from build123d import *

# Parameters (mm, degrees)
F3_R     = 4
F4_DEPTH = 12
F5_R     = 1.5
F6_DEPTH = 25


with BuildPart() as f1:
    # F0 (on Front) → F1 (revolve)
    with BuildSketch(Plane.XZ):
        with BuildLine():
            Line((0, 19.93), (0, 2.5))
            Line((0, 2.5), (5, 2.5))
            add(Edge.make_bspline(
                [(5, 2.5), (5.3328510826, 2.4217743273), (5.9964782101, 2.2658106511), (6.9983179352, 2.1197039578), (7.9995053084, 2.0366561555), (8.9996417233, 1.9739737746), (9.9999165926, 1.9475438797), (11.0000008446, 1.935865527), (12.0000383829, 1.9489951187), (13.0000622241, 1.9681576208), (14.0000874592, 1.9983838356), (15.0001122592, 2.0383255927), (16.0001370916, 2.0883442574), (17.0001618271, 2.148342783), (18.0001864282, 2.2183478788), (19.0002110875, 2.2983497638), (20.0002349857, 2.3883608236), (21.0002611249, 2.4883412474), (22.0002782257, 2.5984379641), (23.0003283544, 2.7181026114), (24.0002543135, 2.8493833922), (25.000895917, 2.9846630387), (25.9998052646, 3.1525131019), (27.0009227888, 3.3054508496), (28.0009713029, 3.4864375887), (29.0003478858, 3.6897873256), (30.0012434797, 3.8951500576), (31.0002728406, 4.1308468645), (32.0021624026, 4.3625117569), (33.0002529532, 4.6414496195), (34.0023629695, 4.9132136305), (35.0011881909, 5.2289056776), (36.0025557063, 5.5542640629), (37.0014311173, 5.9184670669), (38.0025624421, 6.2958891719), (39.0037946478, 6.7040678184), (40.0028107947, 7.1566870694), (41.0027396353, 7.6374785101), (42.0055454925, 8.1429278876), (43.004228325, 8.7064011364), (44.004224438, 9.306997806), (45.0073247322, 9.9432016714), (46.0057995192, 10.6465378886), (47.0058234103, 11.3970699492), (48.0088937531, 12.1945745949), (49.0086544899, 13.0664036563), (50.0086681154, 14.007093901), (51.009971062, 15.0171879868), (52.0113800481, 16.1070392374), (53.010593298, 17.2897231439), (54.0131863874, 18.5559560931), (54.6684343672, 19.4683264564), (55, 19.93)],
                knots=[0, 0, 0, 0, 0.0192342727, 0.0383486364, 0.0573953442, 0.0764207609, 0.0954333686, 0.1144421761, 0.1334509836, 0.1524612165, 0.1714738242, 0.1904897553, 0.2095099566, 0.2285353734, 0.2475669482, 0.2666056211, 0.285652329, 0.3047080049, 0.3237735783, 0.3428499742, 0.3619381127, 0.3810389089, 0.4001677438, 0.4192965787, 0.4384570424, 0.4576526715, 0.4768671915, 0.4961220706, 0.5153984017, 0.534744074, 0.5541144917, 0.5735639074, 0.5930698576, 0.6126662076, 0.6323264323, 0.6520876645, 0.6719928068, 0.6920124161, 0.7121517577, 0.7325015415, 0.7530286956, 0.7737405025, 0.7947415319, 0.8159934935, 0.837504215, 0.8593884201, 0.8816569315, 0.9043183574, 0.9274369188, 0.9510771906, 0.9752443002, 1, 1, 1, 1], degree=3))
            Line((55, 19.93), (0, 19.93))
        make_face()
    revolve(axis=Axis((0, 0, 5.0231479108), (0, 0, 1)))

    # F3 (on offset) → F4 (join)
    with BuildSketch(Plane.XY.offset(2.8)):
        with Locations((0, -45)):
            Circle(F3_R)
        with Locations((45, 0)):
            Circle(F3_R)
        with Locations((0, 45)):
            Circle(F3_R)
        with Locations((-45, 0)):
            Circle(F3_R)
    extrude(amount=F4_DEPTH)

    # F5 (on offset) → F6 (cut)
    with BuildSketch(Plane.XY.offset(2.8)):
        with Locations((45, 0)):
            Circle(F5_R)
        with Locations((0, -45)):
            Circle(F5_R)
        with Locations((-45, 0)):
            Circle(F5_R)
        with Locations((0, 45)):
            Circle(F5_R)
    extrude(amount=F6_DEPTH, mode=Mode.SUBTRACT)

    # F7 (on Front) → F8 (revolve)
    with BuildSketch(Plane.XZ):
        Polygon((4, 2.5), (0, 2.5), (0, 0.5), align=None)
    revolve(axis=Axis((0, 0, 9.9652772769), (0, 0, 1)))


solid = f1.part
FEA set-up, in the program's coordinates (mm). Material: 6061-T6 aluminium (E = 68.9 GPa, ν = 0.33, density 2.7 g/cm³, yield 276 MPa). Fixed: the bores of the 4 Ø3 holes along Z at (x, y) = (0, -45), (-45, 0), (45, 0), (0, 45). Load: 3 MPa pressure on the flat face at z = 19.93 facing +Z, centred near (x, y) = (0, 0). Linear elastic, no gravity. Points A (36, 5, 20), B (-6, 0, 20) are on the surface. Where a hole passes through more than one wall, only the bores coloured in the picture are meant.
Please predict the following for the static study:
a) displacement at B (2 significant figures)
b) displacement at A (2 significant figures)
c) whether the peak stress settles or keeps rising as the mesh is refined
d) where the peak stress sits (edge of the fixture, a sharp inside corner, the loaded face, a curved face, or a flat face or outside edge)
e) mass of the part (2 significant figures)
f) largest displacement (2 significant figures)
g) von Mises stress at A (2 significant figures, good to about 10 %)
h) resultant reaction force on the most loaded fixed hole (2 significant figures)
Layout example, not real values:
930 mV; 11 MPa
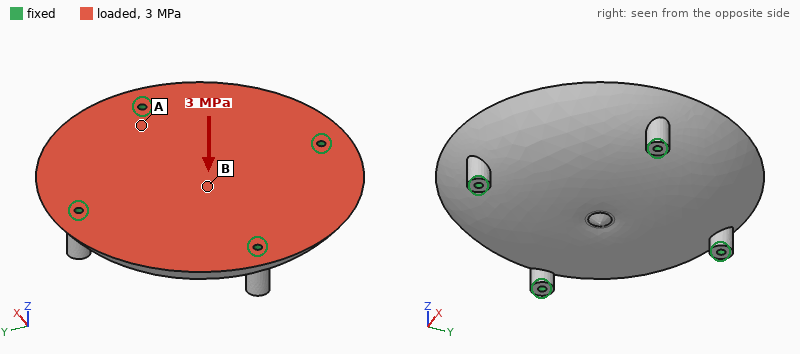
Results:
33 µm; 18 µm; keeps rising; edge of the fixture; 310 g; 46 µm; 30 MPa; 7.2 kN
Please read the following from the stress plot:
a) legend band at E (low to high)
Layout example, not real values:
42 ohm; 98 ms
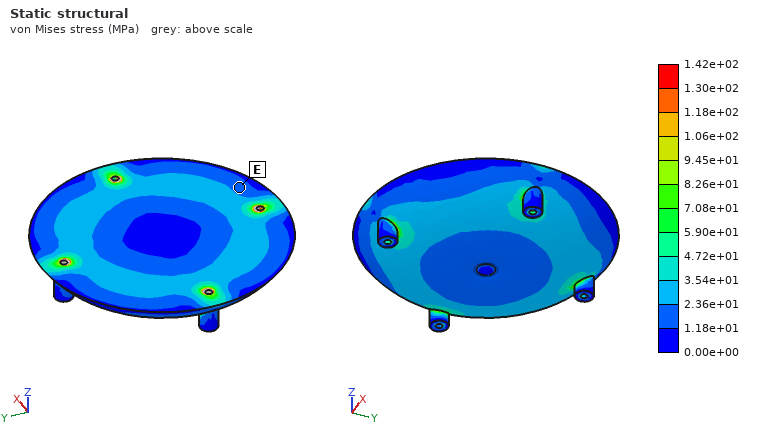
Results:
1.18e+01 to 2.36e+01 MPa
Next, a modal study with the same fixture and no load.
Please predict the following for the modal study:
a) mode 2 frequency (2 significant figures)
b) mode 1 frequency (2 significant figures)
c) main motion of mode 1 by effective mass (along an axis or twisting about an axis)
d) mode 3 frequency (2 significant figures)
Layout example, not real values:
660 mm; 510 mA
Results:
10 kHz; 8400 Hz; along Z; 10 kHz
